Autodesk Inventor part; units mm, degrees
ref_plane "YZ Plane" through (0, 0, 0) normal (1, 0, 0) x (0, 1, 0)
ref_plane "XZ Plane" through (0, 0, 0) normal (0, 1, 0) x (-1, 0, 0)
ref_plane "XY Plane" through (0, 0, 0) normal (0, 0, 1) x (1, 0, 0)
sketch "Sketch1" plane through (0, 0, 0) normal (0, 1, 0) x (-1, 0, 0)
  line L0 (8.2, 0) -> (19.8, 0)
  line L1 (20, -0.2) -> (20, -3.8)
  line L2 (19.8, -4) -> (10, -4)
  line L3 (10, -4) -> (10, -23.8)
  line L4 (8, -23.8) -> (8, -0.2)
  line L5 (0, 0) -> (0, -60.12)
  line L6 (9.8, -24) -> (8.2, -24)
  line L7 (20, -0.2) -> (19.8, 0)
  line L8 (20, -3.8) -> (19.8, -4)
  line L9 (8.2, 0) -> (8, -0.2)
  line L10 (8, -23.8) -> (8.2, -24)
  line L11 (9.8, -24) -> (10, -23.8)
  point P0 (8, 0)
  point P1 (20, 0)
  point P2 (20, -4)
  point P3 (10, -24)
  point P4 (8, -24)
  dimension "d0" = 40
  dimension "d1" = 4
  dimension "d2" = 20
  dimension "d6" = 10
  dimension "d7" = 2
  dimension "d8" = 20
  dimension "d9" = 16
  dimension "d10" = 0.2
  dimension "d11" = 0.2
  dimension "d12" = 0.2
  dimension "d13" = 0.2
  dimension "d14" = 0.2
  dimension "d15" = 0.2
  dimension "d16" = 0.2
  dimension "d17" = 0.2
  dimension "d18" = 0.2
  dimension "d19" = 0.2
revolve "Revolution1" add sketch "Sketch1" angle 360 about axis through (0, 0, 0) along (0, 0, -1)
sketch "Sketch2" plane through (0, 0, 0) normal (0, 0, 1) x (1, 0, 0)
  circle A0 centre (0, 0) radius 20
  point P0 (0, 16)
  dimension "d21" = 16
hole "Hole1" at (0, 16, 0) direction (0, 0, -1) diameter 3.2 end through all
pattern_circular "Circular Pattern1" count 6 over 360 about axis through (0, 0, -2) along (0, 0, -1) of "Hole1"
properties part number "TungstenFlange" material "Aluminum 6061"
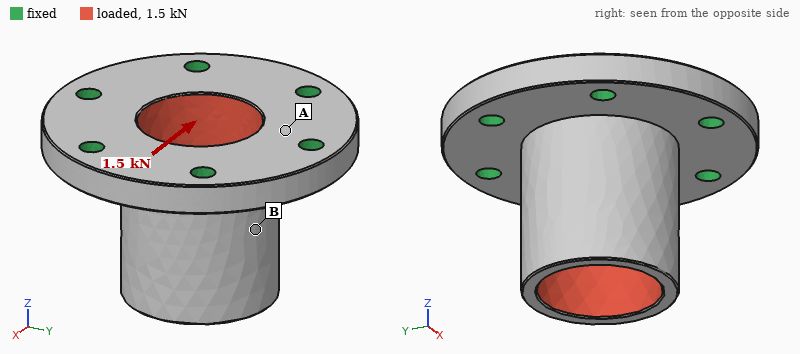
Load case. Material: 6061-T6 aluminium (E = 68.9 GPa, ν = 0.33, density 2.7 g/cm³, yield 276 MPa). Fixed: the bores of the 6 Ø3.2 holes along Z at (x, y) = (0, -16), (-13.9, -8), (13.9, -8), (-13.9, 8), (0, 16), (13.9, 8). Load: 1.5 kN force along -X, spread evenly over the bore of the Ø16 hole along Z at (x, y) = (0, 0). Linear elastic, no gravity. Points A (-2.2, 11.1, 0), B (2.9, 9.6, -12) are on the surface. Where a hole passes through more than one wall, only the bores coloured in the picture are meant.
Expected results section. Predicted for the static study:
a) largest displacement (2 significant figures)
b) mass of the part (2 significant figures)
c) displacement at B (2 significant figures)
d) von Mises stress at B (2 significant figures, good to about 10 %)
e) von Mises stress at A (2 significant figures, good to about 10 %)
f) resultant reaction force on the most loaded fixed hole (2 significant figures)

27 µm
17 g
12 µm
19 MPa
10.0 MPa
460 N
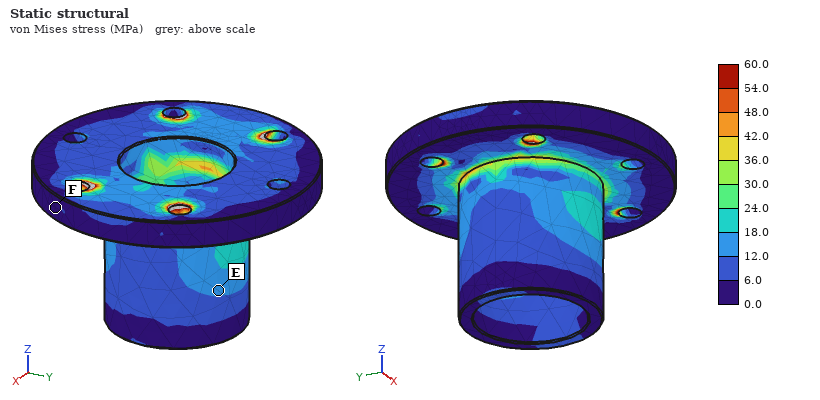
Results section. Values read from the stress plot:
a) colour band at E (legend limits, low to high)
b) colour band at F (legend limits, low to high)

12.0 to 18.0 MPa
0.0 to 6.0 MPa
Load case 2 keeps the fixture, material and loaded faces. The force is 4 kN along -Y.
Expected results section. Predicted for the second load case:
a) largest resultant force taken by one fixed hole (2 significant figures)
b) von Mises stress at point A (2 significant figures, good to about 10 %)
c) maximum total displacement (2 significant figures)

1.4 kN
29 MPa
71 µm
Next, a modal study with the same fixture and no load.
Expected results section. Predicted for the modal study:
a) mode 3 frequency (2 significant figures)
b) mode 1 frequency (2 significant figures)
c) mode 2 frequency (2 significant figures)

19 kHz
16 kHz
16 kHz
